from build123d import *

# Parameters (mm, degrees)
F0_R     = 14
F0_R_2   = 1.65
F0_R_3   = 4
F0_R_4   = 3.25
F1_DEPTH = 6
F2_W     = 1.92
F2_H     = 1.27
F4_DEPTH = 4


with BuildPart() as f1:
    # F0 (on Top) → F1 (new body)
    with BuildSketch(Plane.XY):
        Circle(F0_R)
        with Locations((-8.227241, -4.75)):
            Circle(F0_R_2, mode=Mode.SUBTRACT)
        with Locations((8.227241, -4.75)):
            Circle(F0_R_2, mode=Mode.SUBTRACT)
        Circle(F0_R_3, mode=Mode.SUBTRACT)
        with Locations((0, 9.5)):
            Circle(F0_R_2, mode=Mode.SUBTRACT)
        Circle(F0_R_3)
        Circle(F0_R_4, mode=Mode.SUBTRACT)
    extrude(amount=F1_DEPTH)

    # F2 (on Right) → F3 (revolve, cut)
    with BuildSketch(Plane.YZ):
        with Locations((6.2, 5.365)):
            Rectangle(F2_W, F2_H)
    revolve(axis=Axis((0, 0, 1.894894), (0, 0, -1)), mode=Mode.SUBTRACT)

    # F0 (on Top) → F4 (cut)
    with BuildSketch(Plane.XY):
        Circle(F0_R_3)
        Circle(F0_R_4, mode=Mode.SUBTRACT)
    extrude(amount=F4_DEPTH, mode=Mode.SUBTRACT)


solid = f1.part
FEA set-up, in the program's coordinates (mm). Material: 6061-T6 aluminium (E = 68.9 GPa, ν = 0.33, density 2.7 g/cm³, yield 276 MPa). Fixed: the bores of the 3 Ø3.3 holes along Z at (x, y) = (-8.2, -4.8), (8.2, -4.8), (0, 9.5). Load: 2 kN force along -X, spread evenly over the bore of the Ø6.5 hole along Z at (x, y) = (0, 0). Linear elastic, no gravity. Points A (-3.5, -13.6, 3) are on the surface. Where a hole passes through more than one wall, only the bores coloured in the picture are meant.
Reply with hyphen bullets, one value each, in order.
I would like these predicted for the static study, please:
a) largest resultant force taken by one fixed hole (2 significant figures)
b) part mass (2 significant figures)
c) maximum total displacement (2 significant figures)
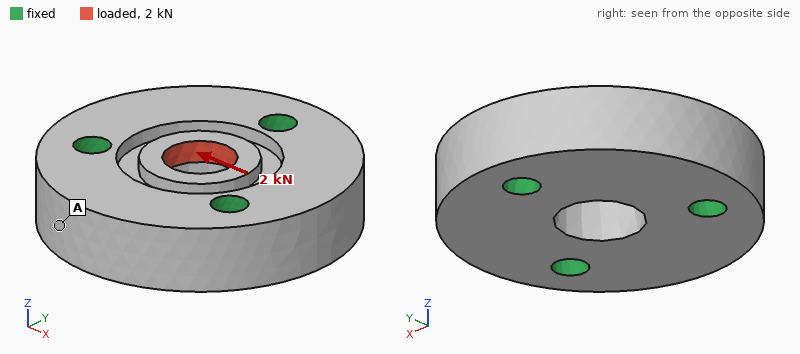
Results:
- 690 N
- 8.6 g
- 8.8 µm
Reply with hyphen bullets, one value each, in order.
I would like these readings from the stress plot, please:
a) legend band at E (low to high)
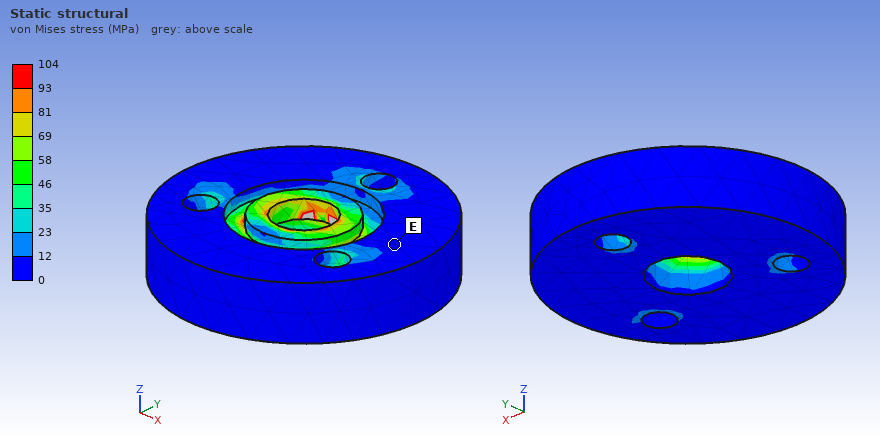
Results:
- 0 to 12 MPa
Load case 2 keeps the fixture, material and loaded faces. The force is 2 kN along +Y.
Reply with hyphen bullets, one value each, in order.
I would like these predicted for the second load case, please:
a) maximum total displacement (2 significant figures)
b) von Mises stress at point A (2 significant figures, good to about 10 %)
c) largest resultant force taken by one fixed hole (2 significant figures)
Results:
- 9.3 µm
- 7.9 MPa
- 690 N
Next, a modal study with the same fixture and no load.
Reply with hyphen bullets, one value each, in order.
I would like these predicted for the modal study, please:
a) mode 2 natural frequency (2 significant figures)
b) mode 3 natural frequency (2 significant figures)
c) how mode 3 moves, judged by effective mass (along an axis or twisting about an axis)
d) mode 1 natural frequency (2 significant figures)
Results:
- 45 kHz
- 49 kHz
- along Z
- 45 kHz
